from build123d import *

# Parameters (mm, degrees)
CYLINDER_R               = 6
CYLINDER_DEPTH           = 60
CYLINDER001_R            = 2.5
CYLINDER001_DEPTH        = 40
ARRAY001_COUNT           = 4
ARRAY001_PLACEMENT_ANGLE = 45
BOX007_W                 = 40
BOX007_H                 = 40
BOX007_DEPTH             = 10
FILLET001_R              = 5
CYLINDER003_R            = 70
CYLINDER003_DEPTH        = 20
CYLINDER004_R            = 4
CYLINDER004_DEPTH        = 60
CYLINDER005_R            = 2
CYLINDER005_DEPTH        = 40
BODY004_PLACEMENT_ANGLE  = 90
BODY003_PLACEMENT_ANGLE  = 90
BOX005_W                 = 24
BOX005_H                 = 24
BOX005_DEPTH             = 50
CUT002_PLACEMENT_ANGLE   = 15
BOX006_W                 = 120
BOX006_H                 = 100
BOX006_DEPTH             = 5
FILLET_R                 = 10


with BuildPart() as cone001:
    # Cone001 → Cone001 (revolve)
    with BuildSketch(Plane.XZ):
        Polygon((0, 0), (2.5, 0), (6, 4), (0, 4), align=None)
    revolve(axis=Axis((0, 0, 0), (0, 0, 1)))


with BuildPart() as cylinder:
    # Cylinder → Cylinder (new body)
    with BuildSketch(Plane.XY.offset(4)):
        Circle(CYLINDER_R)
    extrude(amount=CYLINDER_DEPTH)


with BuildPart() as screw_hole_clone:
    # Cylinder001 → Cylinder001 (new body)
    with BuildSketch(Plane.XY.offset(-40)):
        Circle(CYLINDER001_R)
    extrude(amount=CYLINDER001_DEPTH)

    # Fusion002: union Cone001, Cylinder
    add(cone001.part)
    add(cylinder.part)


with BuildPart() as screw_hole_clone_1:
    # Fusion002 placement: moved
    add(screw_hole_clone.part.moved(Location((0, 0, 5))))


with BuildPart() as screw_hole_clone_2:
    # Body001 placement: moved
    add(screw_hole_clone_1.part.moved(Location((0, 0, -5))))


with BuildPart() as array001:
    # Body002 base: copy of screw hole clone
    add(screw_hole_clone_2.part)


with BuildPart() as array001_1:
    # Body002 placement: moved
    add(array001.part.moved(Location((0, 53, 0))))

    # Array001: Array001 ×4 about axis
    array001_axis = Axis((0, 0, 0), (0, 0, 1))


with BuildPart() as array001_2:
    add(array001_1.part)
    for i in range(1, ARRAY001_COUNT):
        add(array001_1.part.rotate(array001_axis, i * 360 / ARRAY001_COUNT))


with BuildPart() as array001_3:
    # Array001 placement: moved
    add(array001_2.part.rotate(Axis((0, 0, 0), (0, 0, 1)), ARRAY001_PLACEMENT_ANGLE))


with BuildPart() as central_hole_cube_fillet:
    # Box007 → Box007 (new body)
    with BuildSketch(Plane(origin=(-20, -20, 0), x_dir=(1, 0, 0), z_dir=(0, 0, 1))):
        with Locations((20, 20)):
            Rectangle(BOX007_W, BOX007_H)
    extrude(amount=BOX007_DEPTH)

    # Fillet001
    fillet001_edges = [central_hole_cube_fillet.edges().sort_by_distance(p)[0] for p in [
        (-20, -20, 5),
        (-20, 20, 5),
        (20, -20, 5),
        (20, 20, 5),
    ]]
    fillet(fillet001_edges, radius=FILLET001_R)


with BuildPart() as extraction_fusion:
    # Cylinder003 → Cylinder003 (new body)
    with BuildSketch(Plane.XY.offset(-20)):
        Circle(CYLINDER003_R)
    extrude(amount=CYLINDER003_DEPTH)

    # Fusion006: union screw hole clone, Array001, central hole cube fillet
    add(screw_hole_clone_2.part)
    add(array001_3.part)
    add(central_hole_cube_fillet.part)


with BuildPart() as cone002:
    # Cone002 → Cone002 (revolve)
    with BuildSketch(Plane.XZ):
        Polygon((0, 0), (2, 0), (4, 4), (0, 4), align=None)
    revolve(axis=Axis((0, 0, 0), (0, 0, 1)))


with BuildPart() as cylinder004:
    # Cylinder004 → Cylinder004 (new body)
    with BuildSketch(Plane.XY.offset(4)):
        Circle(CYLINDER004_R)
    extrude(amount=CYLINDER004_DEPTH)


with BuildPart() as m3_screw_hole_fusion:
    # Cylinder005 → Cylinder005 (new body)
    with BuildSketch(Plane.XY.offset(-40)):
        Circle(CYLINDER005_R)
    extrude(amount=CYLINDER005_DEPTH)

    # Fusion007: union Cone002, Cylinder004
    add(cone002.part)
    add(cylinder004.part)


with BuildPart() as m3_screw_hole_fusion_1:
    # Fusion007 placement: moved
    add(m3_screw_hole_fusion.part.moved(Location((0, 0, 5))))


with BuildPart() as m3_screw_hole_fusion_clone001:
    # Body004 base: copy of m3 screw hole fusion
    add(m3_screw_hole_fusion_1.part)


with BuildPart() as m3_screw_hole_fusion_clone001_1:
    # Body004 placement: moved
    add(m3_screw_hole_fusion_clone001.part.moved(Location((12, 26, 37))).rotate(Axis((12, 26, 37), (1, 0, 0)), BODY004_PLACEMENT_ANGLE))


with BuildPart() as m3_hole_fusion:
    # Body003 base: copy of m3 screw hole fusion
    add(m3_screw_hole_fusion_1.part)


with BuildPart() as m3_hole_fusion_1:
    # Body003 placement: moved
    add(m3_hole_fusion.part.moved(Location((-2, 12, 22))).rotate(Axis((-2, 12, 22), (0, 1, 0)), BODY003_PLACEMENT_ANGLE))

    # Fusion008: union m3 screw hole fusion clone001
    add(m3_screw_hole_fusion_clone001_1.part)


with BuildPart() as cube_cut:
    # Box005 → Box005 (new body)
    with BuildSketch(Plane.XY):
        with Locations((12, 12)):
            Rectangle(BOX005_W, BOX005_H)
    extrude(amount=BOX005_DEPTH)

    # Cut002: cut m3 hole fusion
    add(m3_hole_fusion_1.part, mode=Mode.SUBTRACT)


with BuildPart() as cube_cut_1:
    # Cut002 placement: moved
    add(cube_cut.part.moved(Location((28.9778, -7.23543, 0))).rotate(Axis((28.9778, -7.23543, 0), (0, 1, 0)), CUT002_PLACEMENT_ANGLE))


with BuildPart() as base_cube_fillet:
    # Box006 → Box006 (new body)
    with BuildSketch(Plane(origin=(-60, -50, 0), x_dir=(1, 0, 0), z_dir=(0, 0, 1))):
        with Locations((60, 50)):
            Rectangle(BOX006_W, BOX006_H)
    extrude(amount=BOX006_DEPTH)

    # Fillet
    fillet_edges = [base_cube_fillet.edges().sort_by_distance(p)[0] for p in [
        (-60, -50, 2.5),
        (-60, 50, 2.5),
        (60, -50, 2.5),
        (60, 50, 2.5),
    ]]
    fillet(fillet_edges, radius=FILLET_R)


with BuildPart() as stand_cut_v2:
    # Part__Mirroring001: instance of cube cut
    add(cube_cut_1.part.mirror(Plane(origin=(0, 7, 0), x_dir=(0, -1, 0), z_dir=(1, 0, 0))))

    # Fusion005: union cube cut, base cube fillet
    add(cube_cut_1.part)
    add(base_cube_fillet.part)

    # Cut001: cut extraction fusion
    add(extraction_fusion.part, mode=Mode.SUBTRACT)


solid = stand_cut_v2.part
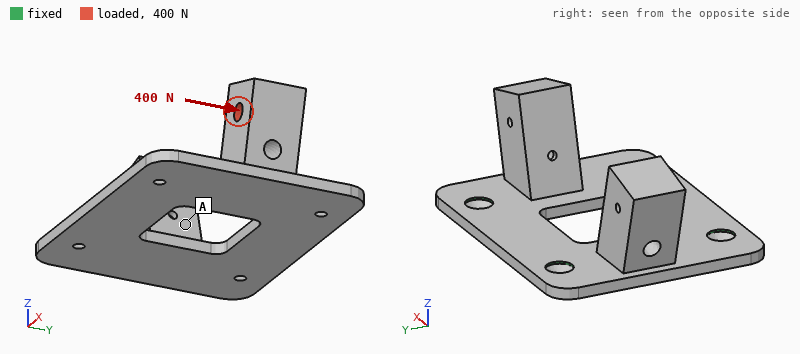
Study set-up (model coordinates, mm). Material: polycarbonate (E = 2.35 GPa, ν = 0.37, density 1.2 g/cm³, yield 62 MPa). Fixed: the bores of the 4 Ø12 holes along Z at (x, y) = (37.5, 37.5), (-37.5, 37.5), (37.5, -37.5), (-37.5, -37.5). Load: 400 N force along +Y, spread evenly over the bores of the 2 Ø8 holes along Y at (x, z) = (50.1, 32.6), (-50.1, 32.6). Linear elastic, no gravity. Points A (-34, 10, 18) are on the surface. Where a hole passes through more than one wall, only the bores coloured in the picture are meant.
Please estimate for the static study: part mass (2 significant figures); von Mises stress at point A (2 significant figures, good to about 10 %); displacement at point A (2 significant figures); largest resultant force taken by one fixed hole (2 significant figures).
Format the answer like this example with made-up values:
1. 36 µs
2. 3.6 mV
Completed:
1. 110 g
2. 1.3 MPa
3. 0.18 mm
4. 170 N
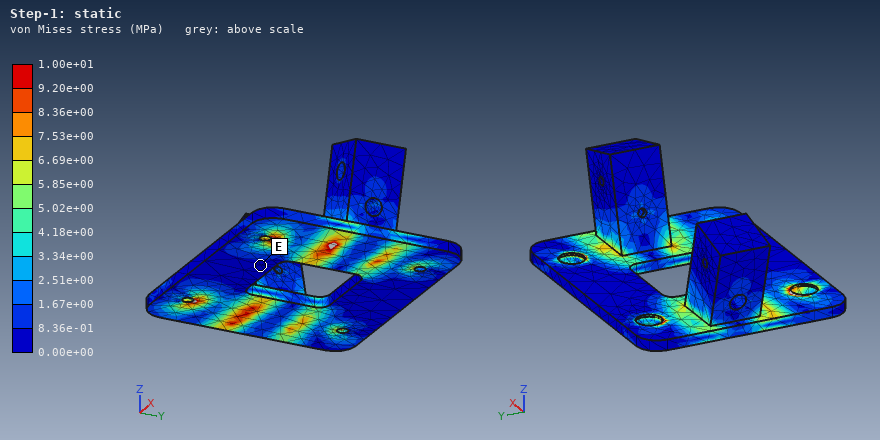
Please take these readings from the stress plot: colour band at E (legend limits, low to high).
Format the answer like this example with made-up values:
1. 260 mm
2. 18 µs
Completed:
1. 0.00e+00 to 8.36e-01 MPa
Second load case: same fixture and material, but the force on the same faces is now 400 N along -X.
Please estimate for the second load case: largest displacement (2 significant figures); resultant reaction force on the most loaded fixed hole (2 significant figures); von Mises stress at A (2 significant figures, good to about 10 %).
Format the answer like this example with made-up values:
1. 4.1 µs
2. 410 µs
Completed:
1. 1.7 mm
2. 120 N
3. 2.6 MPa
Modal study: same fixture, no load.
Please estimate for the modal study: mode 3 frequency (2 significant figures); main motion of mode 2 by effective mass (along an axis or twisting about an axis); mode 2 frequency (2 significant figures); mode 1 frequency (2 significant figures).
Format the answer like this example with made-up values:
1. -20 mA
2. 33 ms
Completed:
1. 710 Hz
2. along X
3. 420 Hz
4. 400 Hz
